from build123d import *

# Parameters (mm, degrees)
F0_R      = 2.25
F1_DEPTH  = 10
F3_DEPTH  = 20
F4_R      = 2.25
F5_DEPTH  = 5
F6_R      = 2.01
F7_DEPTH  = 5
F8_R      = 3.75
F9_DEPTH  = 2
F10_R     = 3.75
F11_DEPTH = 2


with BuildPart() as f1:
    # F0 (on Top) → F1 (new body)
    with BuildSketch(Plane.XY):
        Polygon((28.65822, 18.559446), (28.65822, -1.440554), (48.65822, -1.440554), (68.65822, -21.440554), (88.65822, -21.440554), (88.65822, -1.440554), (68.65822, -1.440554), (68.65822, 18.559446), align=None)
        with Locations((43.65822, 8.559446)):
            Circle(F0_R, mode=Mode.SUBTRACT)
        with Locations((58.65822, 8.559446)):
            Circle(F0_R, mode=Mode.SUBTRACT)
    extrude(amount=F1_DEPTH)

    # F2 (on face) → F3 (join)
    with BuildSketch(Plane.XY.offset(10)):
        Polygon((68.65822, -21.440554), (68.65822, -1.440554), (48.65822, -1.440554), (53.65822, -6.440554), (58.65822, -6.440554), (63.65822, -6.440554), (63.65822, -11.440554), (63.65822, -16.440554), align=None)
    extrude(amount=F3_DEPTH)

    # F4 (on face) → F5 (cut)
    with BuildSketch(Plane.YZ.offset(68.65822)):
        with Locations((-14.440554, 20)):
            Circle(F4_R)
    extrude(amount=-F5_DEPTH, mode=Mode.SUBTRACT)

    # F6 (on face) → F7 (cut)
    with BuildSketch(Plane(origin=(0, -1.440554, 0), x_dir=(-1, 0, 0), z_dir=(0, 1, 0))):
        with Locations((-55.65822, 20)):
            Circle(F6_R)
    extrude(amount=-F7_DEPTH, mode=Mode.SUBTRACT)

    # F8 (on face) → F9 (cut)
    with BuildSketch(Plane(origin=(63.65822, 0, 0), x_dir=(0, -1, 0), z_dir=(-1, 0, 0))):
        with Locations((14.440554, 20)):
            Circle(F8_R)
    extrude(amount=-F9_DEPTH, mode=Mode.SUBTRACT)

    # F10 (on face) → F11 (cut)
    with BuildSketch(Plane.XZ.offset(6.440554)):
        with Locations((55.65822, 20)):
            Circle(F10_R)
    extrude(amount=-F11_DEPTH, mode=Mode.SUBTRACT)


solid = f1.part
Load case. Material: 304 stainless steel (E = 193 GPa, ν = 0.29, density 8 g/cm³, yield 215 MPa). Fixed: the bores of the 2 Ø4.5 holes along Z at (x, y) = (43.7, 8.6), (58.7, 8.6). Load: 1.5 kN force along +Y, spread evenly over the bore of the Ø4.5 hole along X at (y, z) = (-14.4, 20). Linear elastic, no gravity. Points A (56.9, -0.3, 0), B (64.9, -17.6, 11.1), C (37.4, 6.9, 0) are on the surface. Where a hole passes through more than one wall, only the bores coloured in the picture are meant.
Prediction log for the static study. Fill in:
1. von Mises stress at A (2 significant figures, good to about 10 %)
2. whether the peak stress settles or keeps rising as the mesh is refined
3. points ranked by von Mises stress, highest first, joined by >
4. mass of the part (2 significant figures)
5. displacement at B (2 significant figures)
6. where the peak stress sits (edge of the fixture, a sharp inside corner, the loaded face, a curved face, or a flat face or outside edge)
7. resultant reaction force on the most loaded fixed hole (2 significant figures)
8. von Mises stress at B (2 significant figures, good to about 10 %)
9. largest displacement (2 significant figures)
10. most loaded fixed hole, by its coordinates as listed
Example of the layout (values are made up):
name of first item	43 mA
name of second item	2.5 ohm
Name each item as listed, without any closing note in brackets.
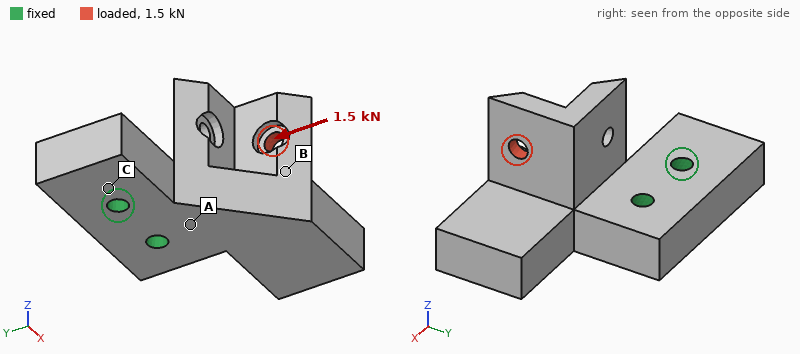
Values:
von Mises stress at A	58 MPa
whether the peak stress settles or keeps rising as the mesh is refined	keeps rising
points ranked by von Mises stress, highest first, joined by >	A > B > C
mass of the part	130 g
displacement at B	27 µm
where the peak stress sits	edge of the fixture
resultant reaction force on the most loaded fixed hole	2.1 kN
von Mises stress at B	43 MPa
largest displacement	52 µm
most loaded fixed hole, by its coordinates as listed	(58.7, 8.6)
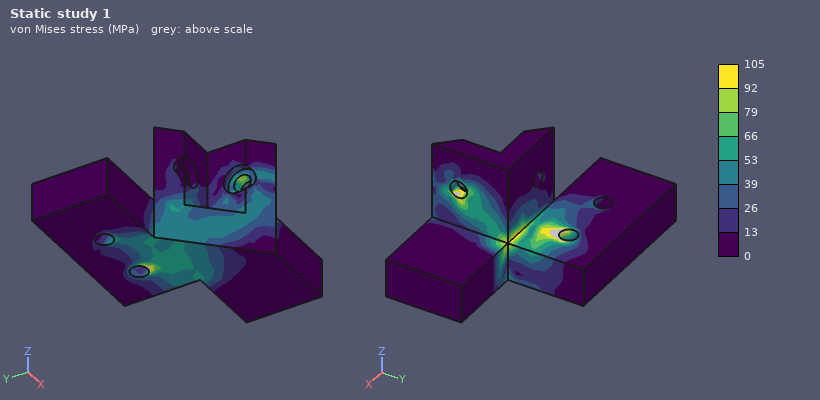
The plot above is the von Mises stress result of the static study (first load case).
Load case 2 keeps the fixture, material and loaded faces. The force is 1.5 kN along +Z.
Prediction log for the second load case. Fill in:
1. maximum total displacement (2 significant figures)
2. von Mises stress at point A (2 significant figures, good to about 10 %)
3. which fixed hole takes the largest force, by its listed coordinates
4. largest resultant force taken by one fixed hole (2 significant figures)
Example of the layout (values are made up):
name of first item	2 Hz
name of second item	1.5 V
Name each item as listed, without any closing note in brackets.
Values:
maximum total displacement	53 µm
von Mises stress at point A	70 MPa
which fixed hole takes the largest force, by its listed coordinates	(58.7, 8.6)
largest resultant force taken by one fixed hole	1.7 kN
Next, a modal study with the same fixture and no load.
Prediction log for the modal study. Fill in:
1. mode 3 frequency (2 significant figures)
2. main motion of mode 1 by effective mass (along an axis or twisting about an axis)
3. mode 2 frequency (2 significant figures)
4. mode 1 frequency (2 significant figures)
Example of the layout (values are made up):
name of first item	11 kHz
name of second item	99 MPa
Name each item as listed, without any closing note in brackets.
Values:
mode 3 frequency	7900 Hz
main motion of mode 1 by effective mass	along Z
mode 2 frequency	6600 Hz
mode 1 frequency	4300 Hz
